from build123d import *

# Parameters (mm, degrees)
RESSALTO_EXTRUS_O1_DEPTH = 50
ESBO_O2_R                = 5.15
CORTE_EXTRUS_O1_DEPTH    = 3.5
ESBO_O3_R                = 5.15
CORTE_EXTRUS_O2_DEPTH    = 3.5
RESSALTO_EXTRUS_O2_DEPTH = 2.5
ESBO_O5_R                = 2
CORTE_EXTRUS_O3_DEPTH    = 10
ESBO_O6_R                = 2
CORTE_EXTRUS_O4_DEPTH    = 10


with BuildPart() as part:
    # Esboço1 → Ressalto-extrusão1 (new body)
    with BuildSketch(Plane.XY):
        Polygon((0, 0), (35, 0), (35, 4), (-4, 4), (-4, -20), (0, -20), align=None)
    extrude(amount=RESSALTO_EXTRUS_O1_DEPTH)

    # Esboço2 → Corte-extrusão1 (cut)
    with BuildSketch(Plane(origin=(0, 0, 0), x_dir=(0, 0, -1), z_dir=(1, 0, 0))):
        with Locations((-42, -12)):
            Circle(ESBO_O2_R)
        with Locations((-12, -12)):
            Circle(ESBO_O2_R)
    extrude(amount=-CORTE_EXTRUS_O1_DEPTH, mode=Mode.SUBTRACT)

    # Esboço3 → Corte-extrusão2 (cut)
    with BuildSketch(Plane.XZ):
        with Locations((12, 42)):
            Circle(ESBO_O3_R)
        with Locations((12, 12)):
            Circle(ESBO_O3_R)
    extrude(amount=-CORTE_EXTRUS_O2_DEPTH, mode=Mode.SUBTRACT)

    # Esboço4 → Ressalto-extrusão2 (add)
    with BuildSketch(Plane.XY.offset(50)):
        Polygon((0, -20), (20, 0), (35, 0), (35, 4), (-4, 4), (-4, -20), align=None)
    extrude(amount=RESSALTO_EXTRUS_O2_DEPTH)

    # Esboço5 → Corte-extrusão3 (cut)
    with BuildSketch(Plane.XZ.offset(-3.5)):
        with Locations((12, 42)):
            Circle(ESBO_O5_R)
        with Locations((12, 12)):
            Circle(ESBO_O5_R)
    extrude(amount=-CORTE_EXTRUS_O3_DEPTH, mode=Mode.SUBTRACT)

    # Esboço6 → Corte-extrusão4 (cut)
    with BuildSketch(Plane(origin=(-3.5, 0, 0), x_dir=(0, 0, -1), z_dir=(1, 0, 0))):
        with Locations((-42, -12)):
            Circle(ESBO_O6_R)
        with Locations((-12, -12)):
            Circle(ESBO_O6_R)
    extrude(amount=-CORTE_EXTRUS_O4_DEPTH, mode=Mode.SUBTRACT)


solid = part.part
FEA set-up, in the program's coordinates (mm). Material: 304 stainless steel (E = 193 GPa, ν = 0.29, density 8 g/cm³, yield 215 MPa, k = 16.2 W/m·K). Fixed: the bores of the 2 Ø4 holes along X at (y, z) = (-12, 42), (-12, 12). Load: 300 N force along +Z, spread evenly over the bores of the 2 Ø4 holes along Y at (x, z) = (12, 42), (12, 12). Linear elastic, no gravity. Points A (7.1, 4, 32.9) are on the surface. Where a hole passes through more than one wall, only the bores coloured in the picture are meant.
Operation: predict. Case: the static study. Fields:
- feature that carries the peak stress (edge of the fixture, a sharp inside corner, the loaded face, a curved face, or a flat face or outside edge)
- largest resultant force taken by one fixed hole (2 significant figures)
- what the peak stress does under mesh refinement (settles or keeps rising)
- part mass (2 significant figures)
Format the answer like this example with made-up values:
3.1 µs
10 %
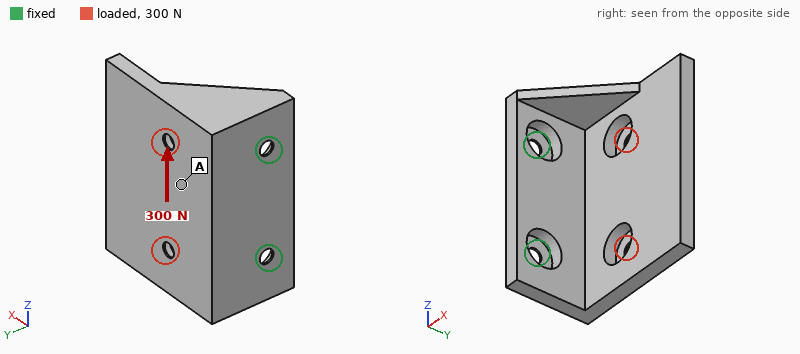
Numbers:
edge of the fixture
270 N
keeps rising
94 g
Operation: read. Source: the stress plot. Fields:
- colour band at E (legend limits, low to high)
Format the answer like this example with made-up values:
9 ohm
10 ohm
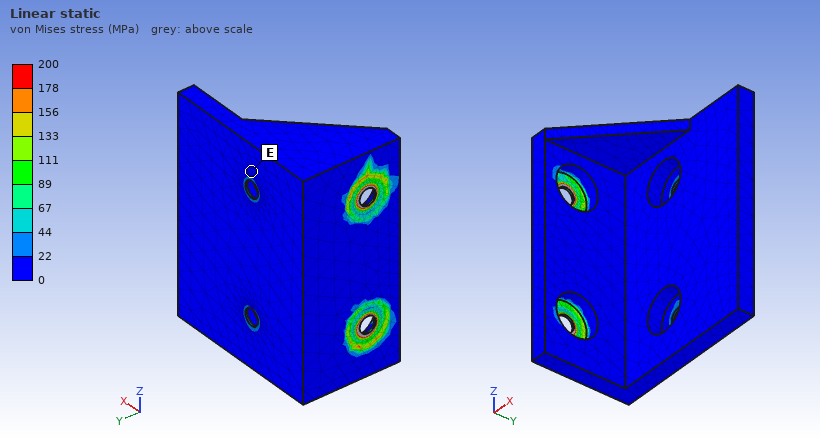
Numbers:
0 to 22 MPa
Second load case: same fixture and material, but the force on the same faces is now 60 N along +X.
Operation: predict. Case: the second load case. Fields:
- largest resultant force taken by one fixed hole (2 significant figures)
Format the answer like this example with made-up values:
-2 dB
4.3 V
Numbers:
31 N
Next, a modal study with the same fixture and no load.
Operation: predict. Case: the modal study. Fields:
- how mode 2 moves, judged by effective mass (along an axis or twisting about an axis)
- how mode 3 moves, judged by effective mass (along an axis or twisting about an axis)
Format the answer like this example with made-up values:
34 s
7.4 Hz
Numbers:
along Z
along X
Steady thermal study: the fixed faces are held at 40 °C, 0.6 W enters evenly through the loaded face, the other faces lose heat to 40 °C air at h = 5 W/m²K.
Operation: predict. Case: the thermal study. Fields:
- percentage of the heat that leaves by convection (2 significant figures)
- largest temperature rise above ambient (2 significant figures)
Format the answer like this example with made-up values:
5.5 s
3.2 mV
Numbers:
37 %
13 K
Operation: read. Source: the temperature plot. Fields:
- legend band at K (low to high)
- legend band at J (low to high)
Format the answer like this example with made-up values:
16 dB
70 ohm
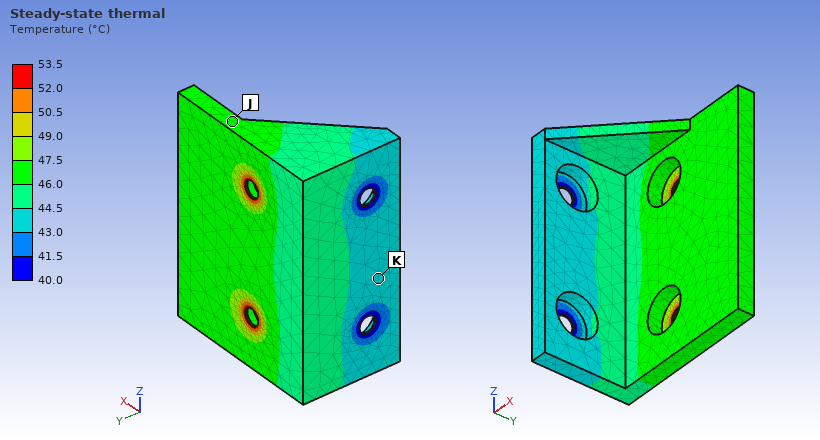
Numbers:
43.0 to 44.5 °C
46.0 to 47.5 °C
